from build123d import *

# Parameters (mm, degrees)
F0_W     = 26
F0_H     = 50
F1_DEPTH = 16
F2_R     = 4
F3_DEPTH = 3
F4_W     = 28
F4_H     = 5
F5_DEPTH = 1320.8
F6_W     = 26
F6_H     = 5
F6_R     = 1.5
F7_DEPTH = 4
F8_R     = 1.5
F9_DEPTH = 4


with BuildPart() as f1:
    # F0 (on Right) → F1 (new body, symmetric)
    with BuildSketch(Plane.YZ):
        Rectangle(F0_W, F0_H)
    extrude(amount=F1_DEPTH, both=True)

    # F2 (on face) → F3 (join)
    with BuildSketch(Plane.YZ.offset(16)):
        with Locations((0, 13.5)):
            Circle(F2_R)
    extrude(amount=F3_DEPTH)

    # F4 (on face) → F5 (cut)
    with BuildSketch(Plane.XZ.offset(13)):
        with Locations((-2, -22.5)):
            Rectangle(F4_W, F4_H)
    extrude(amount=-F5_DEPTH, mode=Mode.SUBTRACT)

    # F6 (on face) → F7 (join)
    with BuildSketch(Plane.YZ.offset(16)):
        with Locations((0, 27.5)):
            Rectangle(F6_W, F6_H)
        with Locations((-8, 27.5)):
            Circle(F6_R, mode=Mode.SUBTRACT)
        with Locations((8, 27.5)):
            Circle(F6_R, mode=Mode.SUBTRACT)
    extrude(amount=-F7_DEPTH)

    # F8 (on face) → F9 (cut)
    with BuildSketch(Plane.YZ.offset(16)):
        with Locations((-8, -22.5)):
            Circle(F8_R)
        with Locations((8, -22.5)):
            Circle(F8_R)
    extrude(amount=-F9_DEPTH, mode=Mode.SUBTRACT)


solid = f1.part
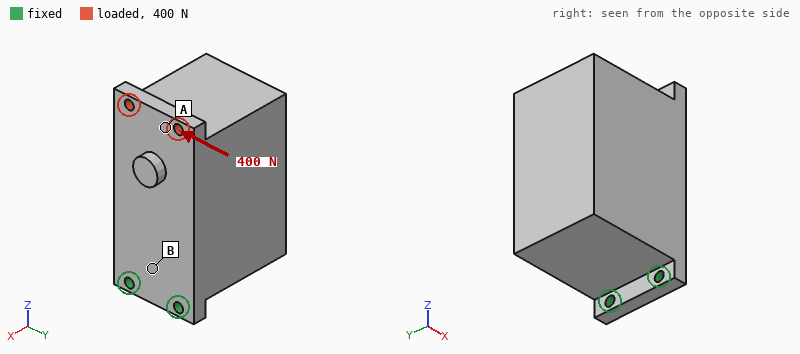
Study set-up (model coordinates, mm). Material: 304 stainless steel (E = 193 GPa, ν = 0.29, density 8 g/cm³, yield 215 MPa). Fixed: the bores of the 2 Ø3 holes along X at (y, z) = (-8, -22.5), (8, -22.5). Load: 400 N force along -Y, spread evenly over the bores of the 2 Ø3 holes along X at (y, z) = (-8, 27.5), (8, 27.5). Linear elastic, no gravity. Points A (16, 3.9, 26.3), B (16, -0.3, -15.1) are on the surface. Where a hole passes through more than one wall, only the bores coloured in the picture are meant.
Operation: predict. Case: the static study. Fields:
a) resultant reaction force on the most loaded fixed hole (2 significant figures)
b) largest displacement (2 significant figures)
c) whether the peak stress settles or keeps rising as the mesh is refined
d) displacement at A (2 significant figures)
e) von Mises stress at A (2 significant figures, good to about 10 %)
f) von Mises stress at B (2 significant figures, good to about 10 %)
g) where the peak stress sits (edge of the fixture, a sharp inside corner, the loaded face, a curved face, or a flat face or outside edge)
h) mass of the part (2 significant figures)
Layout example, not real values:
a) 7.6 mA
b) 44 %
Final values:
a) 1.1 kN
b) 14 µm
c) keeps rising
d) 12 µm
e) 5.8 MPa
f) 16 MPa
g) edge of the fixture
h) 310 g
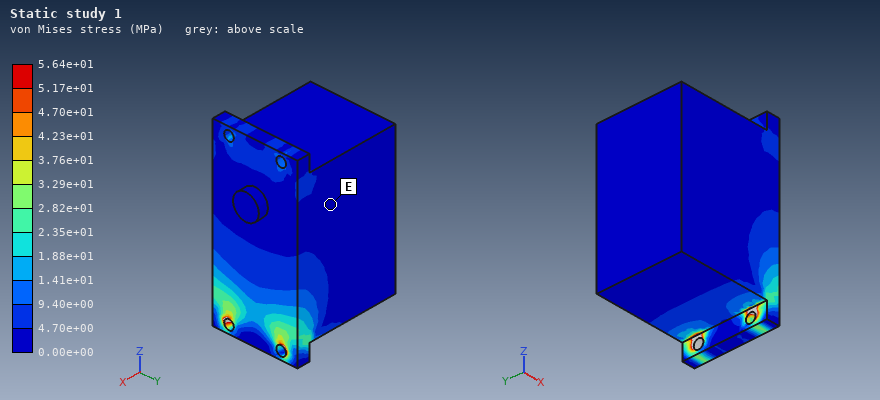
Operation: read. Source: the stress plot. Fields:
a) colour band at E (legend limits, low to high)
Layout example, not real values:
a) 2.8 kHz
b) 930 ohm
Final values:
a) 0.00e+00 to 4.70e+00 MPa
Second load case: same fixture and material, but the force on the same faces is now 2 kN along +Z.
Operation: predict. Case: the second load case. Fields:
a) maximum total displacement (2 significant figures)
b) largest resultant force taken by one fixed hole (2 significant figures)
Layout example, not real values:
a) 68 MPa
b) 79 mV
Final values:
a) 11 µm
b) 1.0 kN
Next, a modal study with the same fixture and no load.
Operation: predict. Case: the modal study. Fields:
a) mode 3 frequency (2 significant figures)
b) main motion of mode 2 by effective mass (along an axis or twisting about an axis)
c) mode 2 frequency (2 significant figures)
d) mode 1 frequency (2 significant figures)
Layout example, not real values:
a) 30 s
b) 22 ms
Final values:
a) 4700 Hz
b) along Y
c) 2900 Hz
d) 660 Hz
